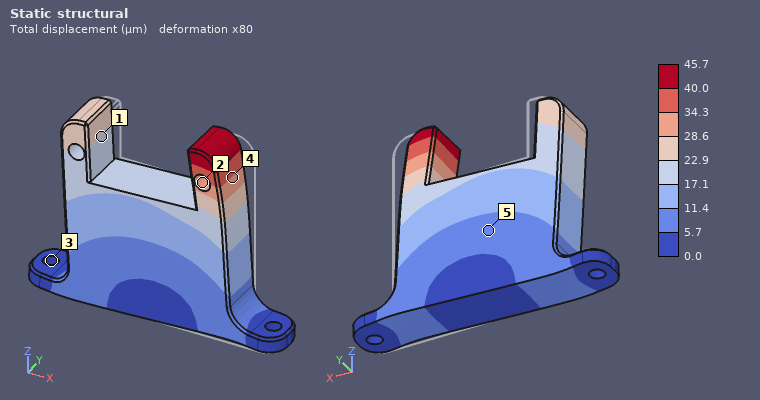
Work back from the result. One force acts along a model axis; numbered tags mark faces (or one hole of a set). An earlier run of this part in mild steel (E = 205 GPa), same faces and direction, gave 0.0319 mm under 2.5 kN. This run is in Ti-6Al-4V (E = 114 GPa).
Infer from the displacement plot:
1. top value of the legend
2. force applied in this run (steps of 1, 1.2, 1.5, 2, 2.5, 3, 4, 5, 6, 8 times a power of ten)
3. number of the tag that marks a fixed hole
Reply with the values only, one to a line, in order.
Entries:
45.7 µm
2 kN
3
